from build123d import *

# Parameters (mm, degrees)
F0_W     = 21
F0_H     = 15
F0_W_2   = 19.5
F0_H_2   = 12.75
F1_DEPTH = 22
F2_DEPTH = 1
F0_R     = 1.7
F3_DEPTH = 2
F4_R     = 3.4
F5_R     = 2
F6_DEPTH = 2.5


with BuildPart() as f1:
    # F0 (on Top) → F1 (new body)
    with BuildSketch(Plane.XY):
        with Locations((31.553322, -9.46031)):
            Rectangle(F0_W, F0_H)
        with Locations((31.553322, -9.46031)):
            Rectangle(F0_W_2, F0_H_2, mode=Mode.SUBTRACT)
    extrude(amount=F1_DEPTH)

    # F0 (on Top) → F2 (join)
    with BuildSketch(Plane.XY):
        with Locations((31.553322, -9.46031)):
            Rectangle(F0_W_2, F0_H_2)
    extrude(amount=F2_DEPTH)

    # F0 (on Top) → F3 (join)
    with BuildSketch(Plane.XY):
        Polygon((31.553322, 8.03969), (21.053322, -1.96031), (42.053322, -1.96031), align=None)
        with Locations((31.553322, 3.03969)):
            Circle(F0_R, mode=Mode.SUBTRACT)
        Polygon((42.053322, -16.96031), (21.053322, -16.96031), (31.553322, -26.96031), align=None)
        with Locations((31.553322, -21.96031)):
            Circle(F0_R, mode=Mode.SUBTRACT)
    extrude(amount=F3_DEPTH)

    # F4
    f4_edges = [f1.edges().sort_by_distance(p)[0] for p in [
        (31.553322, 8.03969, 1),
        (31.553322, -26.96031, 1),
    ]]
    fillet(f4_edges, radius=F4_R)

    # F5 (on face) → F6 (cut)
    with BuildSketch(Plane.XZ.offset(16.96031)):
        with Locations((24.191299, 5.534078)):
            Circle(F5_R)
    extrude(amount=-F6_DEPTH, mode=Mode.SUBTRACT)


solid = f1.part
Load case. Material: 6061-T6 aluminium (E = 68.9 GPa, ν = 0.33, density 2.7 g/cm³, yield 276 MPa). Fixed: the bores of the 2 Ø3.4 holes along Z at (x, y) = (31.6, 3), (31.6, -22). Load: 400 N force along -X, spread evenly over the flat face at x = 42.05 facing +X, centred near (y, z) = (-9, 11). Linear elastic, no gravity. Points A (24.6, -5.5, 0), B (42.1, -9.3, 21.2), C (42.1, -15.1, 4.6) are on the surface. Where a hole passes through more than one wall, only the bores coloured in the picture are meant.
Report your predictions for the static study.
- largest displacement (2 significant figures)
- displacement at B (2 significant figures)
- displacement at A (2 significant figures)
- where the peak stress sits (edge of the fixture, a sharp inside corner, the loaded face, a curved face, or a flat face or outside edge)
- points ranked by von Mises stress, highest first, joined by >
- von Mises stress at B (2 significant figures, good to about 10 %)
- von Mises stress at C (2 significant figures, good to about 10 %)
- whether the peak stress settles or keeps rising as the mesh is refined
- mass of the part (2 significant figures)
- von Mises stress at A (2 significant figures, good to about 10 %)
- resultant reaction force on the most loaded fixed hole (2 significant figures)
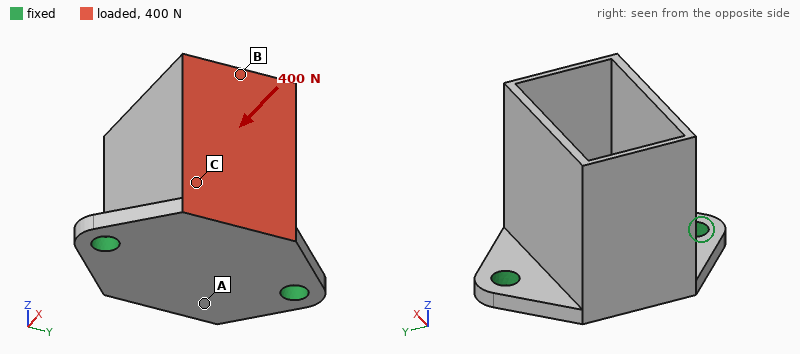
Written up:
0.28 mm
0.27 mm
0.058 mm
edge of the fixture
B > C > A
140 MPa
67 MPa
keeps rising
5.6 g
28 MPa
200 N
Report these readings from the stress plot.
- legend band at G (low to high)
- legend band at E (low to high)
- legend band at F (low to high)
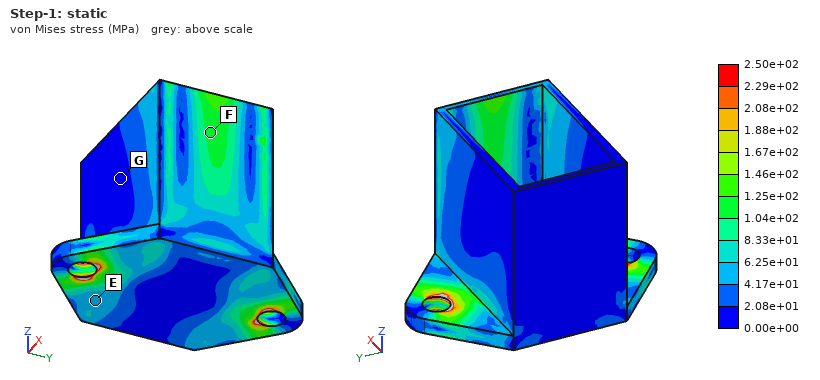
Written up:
0.00e+00 to 2.08e+01 MPa
4.17e+01 to 6.25e+01 MPa
1.04e+02 to 1.25e+02 MPa
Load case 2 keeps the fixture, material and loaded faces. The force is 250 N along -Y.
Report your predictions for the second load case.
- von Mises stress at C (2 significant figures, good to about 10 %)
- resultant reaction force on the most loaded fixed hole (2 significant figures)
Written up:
45 MPa
210 N
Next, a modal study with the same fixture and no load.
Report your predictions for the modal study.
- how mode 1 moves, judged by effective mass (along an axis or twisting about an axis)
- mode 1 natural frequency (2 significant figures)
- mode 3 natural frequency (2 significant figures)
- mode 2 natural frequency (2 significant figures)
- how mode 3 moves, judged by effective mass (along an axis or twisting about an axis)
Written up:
along X
3900 Hz
7600 Hz
6500 Hz
along Y
